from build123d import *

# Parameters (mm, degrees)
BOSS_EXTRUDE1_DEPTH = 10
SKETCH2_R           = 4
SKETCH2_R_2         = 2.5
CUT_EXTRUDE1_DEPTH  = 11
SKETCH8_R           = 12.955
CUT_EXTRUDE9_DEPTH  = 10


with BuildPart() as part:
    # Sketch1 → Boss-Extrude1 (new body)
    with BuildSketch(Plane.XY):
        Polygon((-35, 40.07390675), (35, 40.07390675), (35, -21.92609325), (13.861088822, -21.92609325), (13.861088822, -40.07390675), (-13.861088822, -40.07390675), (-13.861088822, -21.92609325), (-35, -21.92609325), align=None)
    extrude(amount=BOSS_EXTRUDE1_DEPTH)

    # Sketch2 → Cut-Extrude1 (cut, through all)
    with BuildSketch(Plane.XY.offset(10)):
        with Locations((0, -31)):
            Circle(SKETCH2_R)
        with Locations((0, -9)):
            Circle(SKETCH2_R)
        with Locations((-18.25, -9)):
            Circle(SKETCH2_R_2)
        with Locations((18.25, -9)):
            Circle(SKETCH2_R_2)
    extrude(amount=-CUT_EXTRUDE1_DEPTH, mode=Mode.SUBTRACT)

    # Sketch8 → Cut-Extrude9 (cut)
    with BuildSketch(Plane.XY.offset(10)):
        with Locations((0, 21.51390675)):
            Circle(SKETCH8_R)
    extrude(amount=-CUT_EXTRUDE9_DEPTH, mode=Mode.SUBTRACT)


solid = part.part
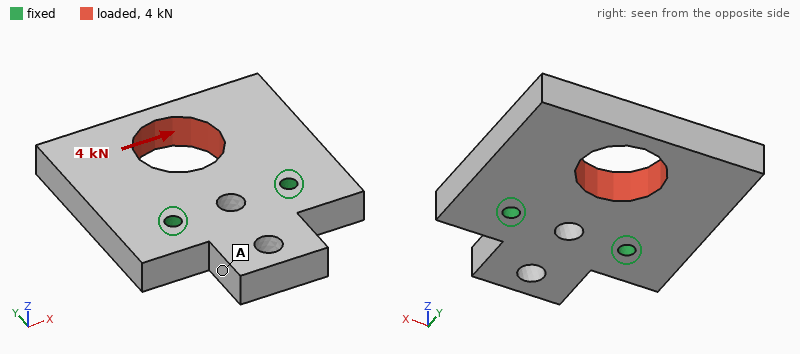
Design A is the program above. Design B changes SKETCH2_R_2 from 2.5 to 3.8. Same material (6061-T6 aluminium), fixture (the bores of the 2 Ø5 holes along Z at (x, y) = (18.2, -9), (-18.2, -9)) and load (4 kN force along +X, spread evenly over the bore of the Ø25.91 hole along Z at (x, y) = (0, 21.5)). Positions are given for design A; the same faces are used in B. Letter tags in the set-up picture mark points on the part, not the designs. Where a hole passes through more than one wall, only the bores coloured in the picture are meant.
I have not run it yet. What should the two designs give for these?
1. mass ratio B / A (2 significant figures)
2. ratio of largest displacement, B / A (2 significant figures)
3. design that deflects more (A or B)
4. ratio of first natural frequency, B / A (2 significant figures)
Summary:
0.99
0.89
A
1.1
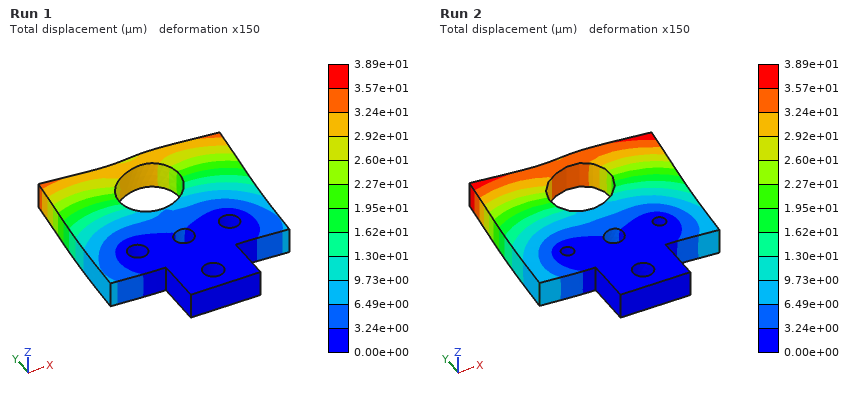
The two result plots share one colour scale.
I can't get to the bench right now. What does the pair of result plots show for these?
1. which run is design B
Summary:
Run 1
